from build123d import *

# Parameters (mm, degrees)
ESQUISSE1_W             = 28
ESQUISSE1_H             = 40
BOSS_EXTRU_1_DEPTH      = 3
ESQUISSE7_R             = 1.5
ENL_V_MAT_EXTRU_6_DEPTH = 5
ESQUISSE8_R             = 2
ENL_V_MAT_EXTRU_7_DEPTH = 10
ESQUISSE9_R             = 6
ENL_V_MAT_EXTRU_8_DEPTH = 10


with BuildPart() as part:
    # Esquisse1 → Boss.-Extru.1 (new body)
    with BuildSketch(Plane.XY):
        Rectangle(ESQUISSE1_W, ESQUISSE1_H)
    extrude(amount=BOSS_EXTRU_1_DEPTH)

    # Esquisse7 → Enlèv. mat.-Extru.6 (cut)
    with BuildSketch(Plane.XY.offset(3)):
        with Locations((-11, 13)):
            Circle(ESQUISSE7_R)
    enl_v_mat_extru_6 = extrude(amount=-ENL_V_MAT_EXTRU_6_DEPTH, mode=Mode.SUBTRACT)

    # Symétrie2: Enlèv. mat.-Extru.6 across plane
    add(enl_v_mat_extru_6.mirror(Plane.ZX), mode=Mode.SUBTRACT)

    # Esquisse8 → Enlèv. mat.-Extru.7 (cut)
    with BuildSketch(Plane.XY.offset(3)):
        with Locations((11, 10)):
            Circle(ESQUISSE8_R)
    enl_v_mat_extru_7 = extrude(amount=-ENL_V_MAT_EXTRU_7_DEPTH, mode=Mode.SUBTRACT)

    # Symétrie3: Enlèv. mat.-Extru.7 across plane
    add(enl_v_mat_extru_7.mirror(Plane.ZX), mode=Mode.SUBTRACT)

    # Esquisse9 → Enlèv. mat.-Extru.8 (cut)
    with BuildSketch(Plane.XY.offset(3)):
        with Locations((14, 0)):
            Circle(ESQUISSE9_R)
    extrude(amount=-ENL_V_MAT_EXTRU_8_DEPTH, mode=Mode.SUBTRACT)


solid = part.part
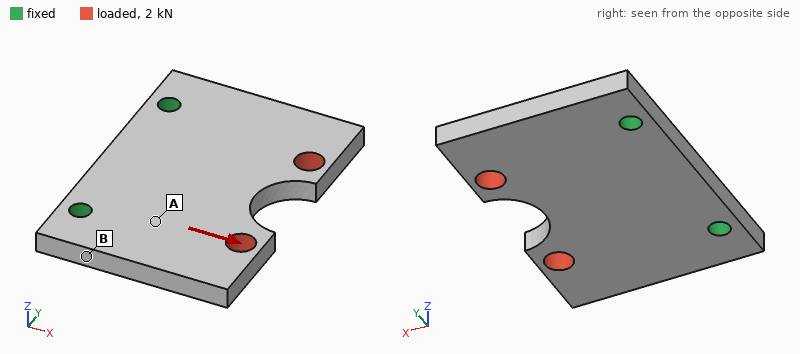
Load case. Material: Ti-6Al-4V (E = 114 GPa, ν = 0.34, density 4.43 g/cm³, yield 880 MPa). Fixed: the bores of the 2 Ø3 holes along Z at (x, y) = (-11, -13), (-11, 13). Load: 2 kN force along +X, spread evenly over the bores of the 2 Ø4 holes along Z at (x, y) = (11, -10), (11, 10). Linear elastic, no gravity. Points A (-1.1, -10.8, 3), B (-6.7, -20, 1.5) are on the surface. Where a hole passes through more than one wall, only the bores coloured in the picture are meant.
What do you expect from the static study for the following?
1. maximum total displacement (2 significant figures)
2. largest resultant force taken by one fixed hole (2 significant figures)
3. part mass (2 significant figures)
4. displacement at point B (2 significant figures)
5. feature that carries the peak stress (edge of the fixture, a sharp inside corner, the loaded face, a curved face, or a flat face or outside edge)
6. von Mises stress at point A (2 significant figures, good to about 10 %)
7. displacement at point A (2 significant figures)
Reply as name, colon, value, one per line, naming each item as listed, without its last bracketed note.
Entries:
maximum total displacement: 9.1 µm
largest resultant force taken by one fixed hole: 1.0 kN
part mass: 14 g
displacement at point B: 2.2 µm
feature that carries the peak stress: a flat face or outside edge
von Mises stress at point A: 26 MPa
displacement at point A: 2.8 µm
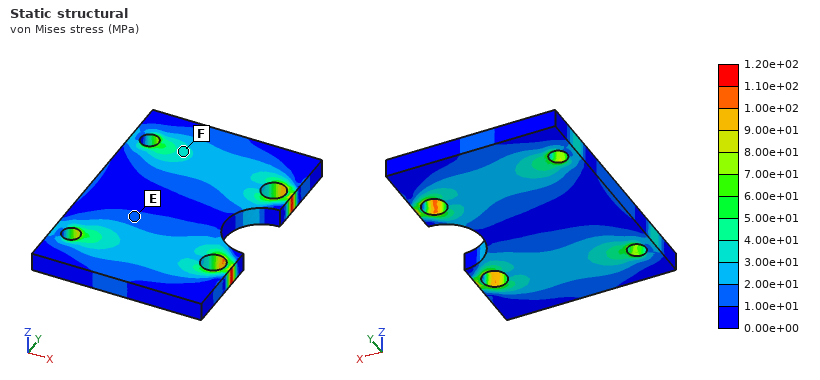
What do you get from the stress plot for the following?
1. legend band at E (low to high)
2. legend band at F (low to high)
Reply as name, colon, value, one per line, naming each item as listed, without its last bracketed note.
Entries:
legend band at E: 1.00e+01 to 2.00e+01 MPa
legend band at F: 3.00e+01 to 4.00e+01 MPa
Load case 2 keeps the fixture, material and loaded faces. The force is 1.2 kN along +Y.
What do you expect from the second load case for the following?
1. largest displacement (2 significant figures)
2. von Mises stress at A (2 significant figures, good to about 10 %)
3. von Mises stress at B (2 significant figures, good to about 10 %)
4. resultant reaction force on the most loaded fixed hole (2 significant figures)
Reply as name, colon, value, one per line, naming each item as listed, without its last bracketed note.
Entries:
largest displacement: 16 µm
von Mises stress at A: 21 MPa
von Mises stress at B: 12 MPa
resultant reaction force on the most loaded fixed hole: 1.1 kN
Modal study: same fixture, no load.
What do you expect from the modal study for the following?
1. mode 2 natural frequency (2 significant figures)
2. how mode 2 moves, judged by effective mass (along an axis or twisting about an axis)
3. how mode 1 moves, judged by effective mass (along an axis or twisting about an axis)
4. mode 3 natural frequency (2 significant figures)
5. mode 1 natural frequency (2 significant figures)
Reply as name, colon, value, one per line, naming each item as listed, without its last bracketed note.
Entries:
mode 2 natural frequency: 6400 Hz
how mode 2 moves, judged by effective mass: twisting about X
how mode 1 moves, judged by effective mass: along Z
mode 3 natural frequency: 13 kHz
mode 1 natural frequency: 4000 Hz
